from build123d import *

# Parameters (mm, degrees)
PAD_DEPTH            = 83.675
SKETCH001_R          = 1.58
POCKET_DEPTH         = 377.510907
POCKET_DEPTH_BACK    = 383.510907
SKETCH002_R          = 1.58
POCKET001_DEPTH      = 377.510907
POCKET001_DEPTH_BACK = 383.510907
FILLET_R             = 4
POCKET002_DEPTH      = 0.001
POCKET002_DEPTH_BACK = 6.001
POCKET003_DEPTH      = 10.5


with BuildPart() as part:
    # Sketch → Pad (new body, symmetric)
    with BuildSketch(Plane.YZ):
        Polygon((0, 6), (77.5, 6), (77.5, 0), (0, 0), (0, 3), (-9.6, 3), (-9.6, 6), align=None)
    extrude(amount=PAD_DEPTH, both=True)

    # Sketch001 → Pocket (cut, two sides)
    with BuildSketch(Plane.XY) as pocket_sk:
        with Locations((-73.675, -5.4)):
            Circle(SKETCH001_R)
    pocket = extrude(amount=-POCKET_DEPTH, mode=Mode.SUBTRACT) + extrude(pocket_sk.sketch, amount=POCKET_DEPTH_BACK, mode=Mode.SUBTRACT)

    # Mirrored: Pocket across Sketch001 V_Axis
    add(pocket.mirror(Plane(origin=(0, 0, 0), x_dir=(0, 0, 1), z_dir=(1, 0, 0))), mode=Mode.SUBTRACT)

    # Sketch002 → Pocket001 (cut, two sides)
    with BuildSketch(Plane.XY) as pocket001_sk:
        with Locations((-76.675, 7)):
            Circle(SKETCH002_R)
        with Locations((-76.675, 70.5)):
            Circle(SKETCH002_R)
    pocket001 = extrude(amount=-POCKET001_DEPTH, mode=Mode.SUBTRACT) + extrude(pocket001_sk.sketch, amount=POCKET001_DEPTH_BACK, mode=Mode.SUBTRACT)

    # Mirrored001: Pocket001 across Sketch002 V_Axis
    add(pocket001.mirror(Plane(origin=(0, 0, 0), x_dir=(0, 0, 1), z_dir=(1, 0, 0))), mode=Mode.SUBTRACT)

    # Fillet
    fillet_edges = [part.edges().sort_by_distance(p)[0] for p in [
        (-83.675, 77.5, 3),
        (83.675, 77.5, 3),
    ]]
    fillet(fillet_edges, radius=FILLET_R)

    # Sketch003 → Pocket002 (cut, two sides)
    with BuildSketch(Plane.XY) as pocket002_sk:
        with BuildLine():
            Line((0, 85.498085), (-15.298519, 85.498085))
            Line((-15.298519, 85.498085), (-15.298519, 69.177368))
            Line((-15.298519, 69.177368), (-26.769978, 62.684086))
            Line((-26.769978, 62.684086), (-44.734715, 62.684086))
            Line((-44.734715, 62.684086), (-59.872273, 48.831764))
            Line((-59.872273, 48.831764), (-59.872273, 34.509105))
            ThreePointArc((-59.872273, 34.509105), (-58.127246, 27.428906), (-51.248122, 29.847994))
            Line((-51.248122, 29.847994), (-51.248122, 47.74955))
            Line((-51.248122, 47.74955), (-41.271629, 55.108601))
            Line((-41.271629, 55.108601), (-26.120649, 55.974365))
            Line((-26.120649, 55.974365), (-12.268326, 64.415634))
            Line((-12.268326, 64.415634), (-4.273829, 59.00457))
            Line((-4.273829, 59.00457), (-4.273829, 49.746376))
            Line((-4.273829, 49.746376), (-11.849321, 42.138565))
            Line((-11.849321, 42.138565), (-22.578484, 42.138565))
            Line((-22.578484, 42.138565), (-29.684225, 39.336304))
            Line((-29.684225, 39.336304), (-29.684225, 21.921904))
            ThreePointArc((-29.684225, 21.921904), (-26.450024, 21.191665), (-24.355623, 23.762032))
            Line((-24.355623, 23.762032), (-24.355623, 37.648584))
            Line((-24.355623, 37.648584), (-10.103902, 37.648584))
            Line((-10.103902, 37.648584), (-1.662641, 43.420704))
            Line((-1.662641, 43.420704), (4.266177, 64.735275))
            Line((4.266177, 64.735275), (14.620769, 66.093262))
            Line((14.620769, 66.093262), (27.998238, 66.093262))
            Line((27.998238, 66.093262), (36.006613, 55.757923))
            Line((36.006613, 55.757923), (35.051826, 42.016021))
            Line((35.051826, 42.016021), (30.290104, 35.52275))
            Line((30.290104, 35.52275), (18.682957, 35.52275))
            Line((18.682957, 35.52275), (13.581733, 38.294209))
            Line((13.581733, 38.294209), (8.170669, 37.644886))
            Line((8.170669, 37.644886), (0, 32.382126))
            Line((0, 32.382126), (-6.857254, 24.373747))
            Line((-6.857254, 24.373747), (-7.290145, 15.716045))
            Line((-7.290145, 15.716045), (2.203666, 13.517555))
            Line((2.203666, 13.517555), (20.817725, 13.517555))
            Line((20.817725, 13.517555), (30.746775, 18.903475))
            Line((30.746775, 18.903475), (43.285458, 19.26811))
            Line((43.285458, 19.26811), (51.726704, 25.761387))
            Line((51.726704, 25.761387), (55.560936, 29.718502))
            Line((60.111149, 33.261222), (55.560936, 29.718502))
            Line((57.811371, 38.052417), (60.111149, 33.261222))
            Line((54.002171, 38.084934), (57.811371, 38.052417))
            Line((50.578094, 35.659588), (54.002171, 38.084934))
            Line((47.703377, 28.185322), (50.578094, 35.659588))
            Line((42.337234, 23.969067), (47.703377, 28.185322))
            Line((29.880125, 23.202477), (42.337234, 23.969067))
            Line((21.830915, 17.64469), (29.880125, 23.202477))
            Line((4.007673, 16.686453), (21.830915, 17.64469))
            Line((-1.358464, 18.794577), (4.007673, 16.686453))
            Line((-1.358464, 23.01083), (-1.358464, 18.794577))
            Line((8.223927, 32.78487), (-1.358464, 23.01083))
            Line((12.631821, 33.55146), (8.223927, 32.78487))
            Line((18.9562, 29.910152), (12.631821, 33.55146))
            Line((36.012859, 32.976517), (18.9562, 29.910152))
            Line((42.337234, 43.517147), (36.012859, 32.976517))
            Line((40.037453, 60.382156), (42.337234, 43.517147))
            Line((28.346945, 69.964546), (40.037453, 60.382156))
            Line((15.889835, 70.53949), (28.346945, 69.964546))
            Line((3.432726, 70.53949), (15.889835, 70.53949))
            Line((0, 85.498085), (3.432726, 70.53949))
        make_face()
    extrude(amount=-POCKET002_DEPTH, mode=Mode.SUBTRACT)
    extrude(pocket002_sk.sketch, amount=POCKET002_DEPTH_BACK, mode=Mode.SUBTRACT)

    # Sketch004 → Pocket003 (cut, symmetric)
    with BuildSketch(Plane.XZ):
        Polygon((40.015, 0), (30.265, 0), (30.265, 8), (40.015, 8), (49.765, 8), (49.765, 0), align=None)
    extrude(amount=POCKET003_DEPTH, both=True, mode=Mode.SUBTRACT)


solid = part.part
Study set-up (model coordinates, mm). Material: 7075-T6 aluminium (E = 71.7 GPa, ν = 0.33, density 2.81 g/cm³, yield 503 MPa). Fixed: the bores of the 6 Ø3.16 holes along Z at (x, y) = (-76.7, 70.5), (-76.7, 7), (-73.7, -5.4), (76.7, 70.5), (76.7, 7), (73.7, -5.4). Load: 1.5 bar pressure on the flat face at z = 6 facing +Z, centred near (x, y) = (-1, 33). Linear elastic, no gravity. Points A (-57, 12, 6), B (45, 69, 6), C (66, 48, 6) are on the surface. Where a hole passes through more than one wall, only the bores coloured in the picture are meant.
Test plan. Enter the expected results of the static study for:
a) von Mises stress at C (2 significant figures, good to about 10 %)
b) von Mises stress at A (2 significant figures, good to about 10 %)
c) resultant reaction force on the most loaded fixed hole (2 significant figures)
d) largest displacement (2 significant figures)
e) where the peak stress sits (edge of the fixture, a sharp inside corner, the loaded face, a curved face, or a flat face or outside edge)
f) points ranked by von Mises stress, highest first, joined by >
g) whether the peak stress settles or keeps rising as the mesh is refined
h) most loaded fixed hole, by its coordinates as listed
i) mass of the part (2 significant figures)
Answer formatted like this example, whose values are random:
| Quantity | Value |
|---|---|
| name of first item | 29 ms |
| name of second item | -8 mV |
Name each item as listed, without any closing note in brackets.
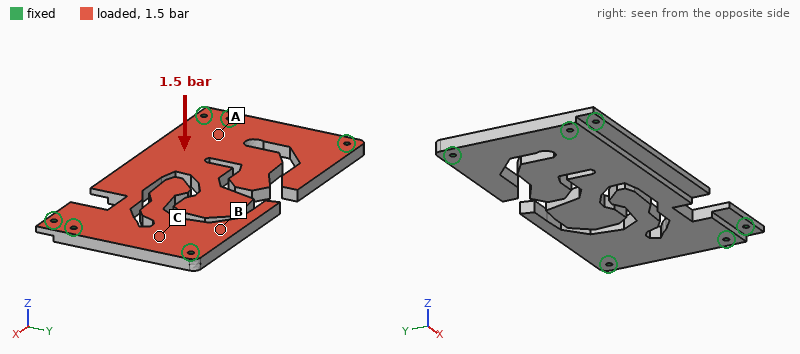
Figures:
| Quantity | Value |
|---|---|
| von Mises stress at C | 27 MPa |
| von Mises stress at A | 47 MPa |
| resultant reaction force on the most loaded fixed hole | 870 N |
| largest displacement | 1.7 mm |
| where the peak stress sits | edge of the fixture |
| points ranked by von Mises stress, highest first, joined by > | A > C > B |
| whether the peak stress settles or keeps rising as the mesh is refined | keeps rising |
| most loaded fixed hole, by its coordinates as listed | (-76.7, 7) |
| mass of the part | 190 g |
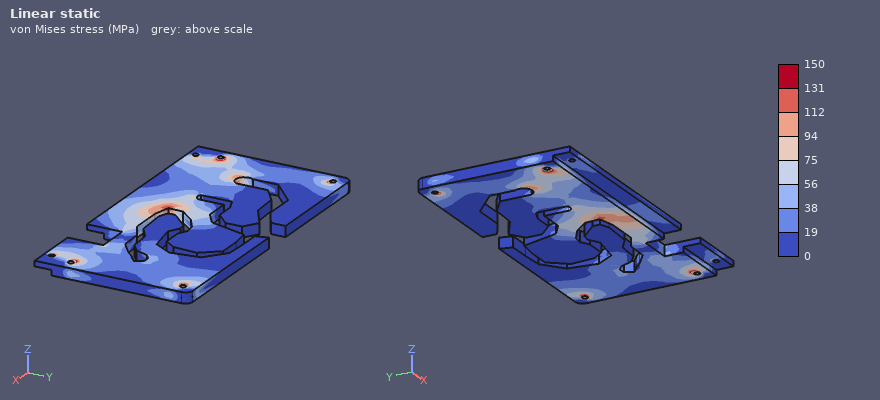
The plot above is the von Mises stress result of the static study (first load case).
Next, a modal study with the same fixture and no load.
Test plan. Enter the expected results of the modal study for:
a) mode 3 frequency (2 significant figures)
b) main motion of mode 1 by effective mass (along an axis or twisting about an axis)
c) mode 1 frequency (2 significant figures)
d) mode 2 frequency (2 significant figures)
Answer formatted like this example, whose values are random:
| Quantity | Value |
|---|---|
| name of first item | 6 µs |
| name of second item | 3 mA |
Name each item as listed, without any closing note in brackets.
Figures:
| Quantity | Value |
|---|---|
| mode 3 frequency | 1100 Hz |
| main motion of mode 1 by effective mass | along Z |
| mode 1 frequency | 490 Hz |
| mode 2 frequency | 890 Hz |
